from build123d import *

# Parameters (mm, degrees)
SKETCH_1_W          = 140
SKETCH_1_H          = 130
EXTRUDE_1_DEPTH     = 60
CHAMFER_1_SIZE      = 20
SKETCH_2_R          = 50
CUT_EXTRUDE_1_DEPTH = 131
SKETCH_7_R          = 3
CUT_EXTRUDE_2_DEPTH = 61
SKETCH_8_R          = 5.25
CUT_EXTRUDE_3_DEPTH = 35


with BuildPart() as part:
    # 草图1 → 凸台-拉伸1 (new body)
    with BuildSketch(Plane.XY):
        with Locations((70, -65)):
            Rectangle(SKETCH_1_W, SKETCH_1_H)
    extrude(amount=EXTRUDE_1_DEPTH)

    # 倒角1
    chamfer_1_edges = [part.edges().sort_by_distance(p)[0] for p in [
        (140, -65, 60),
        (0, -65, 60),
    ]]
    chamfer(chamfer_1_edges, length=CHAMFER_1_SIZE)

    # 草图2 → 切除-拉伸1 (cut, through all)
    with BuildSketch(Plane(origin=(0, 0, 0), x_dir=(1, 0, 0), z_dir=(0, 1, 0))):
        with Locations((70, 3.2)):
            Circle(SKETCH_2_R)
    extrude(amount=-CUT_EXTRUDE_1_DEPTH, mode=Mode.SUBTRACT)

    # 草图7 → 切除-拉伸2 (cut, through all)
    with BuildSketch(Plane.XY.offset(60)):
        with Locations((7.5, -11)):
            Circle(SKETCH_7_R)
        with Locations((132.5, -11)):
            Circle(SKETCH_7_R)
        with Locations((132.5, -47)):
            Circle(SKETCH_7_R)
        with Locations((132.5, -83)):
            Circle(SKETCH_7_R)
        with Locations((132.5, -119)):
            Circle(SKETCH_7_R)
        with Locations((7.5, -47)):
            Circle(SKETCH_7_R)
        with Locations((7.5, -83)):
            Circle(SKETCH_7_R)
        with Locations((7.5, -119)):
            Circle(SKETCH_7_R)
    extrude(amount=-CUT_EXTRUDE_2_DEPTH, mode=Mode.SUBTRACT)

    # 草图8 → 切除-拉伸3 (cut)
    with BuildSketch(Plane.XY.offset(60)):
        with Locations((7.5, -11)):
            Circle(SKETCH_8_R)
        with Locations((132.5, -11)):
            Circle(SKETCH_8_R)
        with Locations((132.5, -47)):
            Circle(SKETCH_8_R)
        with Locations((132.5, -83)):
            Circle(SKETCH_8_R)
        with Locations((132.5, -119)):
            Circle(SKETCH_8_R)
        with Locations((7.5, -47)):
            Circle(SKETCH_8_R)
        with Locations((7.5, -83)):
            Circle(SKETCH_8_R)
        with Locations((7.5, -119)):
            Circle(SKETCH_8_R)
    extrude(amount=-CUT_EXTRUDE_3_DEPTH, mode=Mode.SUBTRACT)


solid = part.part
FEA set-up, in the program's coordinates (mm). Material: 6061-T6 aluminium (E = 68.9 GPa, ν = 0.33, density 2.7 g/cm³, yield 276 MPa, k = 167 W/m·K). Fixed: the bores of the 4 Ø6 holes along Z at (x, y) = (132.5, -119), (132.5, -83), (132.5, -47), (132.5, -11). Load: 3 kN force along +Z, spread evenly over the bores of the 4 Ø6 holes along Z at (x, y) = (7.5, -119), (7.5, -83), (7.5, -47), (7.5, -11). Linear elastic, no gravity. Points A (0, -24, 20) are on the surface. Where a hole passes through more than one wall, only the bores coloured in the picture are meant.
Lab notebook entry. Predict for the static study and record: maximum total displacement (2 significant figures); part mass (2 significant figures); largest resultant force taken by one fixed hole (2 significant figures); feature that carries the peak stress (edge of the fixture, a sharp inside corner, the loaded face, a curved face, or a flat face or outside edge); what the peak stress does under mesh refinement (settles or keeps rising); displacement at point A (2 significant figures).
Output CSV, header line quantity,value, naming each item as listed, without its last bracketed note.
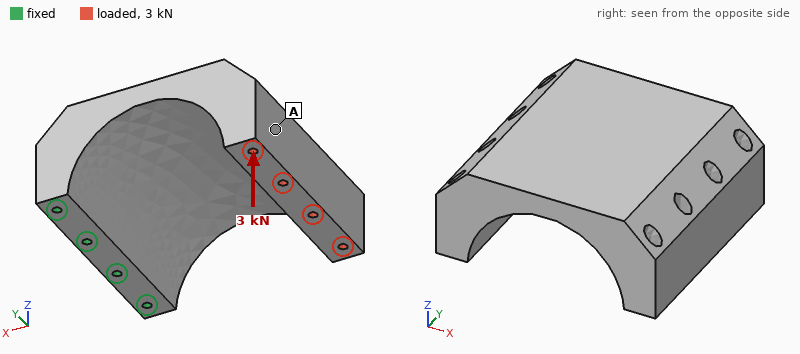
quantity,value
maximum total displacement,0.55 mm
part mass,1.5 kg
largest resultant force taken by one fixed hole,1.4 kN
feature that carries the peak stress,edge of the fixture
what the peak stress does under mesh refinement,keeps rising
displacement at point A,0.51 mm
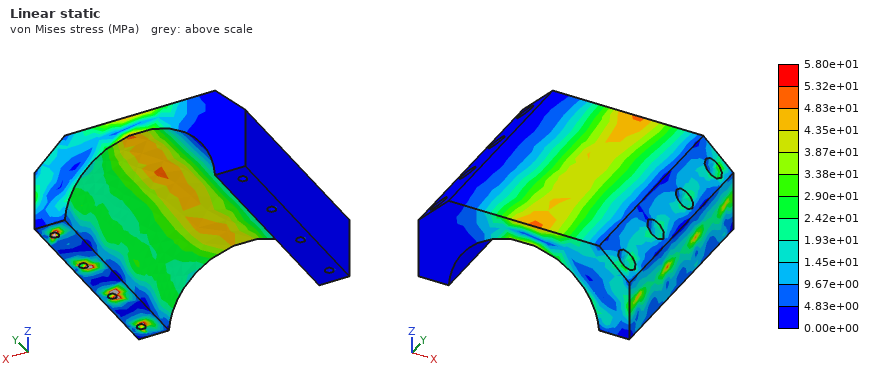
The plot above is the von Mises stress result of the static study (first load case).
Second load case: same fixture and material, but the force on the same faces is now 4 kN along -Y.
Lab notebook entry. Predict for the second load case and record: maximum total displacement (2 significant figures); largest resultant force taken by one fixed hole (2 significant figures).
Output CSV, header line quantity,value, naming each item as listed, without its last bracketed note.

quantity,value
maximum total displacement,0.20 mm
largest resultant force taken by one fixed hole,4.2 kN
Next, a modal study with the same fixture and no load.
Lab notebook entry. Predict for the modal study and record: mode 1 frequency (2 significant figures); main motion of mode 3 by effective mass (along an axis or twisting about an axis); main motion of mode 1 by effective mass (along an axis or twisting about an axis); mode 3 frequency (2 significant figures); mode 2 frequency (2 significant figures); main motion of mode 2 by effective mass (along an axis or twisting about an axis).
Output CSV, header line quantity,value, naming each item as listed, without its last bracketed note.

quantity,value
mode 1 frequency,580 Hz
main motion of mode 3 by effective mass,along X
main motion of mode 1 by effective mass,along Z
mode 3 frequency,1900 Hz
mode 2 frequency,1200 Hz
main motion of mode 2 by effective mass,along Y
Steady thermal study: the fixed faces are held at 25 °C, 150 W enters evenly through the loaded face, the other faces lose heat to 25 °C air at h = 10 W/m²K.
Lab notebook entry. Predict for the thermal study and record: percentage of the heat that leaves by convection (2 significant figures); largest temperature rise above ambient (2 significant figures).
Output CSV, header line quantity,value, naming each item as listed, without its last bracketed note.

quantity,value
percentage of the heat that leaves by convection,11 %
largest temperature rise above ambient,52 K
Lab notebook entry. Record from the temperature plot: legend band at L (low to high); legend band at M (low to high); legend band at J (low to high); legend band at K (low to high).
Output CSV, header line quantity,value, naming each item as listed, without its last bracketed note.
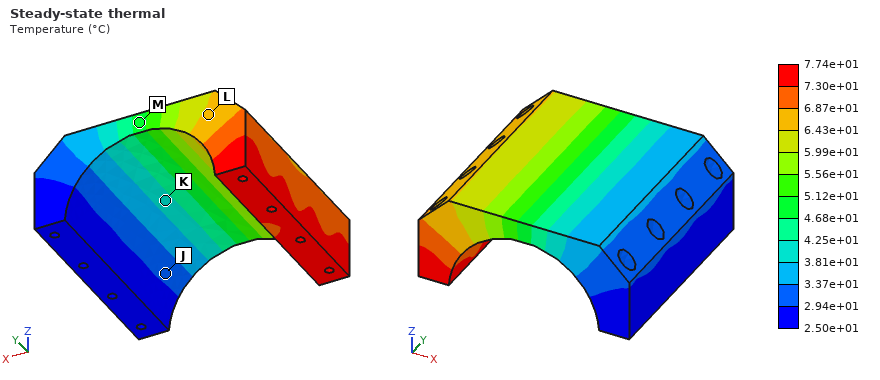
quantity,value
legend band at L,6.43e+01 to 6.87e+01 °C
legend band at M,4.68e+01 to 5.12e+01 °C
legend band at J,2.94e+01 to 3.37e+01 °C
legend band at K,3.81e+01 to 4.25e+01 °C
